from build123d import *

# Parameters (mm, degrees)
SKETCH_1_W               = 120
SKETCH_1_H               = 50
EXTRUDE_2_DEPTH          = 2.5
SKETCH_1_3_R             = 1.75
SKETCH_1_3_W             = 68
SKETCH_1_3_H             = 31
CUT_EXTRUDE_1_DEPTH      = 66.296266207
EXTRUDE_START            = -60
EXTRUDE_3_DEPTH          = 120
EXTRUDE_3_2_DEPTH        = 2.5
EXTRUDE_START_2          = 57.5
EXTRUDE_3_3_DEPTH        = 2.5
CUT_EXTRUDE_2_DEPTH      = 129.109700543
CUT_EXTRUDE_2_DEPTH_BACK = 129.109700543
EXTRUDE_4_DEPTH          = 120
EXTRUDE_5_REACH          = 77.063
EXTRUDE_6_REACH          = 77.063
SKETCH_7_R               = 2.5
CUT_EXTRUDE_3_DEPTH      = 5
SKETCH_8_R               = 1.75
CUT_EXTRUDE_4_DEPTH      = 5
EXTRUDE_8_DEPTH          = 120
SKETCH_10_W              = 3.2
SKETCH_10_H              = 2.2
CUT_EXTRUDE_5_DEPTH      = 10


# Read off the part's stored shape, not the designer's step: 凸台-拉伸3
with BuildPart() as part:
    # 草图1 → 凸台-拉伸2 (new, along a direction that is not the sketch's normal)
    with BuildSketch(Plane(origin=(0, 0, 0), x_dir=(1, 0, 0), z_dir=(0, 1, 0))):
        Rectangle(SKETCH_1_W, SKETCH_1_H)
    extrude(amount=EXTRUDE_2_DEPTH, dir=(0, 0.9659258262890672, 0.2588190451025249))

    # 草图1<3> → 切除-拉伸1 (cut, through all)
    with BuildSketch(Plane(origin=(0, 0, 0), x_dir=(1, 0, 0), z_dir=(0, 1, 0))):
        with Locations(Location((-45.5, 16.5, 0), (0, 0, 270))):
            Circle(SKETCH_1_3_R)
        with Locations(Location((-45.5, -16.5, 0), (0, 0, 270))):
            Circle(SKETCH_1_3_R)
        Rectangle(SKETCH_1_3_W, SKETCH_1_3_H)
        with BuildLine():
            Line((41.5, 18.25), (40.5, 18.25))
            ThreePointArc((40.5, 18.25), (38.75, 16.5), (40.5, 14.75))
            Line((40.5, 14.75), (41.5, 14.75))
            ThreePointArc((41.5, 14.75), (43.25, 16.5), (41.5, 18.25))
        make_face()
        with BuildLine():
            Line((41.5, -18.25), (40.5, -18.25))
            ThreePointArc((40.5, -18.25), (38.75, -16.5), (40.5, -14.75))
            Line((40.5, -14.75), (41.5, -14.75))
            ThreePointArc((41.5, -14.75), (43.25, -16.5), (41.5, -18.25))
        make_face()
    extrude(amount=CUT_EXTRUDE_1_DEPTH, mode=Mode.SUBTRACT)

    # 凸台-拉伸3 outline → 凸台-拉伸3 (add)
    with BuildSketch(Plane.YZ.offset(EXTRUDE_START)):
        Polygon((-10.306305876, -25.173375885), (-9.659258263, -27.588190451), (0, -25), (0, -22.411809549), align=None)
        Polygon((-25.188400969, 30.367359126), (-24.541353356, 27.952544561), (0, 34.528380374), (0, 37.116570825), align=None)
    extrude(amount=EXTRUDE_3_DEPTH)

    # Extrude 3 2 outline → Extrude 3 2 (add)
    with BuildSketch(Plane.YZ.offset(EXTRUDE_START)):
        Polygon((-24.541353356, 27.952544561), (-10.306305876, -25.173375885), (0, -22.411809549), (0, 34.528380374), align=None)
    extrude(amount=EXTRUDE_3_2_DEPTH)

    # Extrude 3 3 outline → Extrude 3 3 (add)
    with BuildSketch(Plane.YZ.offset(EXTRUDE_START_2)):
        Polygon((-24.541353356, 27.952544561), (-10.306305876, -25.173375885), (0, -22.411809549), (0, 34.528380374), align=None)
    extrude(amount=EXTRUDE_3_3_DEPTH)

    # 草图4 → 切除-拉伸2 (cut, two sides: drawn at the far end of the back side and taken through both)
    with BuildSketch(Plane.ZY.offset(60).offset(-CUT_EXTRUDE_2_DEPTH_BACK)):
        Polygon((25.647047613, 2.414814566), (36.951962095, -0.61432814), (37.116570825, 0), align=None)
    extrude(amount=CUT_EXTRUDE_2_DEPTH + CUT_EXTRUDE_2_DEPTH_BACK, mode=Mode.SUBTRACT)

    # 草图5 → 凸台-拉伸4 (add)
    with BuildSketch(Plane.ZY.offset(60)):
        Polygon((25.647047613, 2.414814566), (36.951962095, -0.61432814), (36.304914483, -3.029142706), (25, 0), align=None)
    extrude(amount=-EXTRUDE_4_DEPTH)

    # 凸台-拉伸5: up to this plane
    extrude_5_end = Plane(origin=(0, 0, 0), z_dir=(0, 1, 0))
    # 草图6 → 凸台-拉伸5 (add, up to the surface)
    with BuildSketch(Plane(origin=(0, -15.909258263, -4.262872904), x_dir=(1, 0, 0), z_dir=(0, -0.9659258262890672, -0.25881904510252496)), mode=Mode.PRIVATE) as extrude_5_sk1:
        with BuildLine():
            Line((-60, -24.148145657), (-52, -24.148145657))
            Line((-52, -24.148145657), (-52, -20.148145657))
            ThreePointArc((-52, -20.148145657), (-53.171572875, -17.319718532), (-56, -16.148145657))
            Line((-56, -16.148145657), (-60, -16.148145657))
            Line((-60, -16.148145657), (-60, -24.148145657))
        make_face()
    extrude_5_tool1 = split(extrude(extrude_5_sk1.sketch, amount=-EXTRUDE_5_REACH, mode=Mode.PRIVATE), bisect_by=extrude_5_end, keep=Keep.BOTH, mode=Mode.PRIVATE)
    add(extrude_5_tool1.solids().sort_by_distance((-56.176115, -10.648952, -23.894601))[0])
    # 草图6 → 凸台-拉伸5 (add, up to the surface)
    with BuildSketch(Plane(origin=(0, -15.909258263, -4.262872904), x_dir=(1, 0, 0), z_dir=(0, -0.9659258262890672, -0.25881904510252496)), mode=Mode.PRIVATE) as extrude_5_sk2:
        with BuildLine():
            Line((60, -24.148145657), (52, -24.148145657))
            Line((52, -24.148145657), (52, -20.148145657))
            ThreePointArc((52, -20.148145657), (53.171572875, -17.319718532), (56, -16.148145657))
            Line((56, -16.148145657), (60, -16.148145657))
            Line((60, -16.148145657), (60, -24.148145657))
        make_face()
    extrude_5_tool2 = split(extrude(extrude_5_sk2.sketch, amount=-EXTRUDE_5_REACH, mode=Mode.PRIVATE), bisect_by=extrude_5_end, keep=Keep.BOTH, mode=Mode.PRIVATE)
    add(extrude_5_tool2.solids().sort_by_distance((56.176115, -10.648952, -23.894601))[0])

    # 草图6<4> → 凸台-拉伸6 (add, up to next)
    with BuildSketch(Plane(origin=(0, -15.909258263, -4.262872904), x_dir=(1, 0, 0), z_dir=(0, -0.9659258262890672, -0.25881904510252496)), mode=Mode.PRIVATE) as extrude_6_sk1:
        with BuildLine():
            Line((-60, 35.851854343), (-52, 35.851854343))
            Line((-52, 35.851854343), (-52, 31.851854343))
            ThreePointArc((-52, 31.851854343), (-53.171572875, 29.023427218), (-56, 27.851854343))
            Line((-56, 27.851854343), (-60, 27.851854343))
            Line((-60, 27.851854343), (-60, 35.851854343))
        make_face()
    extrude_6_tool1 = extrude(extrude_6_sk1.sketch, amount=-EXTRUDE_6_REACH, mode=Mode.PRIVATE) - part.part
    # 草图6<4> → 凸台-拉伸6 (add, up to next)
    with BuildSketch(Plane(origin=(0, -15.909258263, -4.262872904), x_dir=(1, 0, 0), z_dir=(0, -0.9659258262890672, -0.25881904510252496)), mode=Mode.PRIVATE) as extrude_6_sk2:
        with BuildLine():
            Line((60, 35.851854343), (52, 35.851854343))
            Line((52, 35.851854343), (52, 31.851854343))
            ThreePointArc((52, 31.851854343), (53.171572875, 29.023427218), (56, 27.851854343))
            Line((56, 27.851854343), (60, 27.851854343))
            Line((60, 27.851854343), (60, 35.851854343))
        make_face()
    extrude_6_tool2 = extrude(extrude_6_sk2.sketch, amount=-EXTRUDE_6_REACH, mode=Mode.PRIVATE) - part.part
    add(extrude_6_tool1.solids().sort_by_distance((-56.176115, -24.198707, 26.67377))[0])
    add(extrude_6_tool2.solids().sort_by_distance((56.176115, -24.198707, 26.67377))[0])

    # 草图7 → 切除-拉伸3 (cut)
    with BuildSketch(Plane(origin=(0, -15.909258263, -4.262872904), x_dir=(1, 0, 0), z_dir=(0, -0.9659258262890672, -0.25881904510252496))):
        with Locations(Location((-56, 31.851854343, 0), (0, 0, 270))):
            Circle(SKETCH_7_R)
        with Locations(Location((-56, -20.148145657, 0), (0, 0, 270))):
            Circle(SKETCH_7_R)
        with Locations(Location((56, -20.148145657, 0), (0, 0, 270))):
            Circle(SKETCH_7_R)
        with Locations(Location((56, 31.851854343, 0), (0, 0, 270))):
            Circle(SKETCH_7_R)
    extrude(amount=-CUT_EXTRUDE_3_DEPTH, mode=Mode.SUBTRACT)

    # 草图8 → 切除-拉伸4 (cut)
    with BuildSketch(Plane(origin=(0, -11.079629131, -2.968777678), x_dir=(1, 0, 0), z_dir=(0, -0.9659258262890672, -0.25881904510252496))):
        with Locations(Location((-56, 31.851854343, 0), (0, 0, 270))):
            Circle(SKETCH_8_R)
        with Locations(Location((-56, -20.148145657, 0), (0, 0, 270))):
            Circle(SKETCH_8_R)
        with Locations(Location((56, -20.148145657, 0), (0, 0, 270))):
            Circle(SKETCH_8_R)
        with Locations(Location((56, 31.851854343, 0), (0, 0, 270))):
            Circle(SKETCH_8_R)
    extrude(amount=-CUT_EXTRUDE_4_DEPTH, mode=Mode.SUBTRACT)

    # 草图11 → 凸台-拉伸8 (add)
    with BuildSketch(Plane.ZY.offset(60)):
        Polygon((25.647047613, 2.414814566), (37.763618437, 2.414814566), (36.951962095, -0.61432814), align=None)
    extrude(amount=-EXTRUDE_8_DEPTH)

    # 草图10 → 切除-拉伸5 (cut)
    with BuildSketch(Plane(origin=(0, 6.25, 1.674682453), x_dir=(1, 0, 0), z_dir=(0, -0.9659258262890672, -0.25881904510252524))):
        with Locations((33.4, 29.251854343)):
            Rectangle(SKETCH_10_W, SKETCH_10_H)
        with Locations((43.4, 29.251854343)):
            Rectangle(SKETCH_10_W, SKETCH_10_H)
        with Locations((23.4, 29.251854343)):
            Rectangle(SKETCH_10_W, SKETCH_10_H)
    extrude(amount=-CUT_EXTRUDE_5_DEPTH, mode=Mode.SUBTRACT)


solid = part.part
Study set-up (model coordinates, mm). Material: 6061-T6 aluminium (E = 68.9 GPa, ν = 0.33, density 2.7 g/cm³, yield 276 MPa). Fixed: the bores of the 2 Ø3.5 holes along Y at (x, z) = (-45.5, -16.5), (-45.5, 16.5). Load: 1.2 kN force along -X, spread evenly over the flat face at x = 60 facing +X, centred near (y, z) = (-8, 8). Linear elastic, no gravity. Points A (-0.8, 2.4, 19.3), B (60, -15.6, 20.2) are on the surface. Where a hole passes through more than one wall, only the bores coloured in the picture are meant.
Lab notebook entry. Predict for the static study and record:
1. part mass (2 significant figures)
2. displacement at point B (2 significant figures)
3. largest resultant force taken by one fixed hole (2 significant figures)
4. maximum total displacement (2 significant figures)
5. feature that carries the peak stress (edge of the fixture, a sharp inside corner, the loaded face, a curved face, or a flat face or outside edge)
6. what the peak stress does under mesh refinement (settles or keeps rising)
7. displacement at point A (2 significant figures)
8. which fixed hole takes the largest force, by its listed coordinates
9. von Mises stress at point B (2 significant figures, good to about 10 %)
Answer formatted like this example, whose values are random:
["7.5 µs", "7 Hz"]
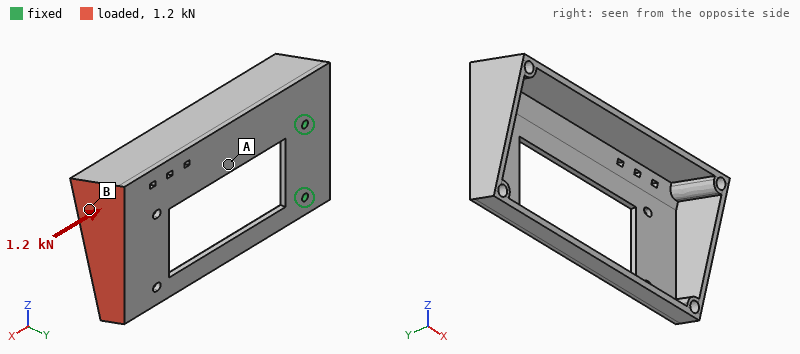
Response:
["84 g", "1.5 mm", "880 N", "1.5 mm", "edge of the fixture", "keeps rising", "0.57 mm", "(-45.5, 16.5)", "35 MPa"]
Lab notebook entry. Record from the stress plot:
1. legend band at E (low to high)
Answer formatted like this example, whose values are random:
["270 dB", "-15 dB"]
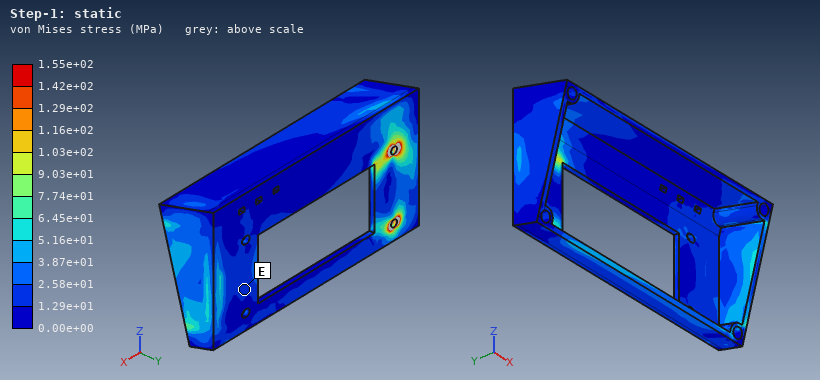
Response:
["1.29e+01 to 2.58e+01 MPa"]
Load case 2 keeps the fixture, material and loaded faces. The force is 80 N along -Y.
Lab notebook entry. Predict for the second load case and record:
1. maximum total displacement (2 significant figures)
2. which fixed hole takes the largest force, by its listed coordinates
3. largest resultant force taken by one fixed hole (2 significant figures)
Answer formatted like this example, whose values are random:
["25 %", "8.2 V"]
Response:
["1.1 mm", "(-45.5, 16.5)", "73 N"]
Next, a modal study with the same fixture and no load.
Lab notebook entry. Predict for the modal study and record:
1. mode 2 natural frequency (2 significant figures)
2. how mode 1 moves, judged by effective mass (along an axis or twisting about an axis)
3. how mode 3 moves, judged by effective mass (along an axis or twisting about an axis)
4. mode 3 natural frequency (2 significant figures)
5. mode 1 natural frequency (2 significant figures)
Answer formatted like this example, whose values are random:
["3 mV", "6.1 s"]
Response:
["600 Hz", "along Y", "along Z", "1200 Hz", "260 Hz"]
